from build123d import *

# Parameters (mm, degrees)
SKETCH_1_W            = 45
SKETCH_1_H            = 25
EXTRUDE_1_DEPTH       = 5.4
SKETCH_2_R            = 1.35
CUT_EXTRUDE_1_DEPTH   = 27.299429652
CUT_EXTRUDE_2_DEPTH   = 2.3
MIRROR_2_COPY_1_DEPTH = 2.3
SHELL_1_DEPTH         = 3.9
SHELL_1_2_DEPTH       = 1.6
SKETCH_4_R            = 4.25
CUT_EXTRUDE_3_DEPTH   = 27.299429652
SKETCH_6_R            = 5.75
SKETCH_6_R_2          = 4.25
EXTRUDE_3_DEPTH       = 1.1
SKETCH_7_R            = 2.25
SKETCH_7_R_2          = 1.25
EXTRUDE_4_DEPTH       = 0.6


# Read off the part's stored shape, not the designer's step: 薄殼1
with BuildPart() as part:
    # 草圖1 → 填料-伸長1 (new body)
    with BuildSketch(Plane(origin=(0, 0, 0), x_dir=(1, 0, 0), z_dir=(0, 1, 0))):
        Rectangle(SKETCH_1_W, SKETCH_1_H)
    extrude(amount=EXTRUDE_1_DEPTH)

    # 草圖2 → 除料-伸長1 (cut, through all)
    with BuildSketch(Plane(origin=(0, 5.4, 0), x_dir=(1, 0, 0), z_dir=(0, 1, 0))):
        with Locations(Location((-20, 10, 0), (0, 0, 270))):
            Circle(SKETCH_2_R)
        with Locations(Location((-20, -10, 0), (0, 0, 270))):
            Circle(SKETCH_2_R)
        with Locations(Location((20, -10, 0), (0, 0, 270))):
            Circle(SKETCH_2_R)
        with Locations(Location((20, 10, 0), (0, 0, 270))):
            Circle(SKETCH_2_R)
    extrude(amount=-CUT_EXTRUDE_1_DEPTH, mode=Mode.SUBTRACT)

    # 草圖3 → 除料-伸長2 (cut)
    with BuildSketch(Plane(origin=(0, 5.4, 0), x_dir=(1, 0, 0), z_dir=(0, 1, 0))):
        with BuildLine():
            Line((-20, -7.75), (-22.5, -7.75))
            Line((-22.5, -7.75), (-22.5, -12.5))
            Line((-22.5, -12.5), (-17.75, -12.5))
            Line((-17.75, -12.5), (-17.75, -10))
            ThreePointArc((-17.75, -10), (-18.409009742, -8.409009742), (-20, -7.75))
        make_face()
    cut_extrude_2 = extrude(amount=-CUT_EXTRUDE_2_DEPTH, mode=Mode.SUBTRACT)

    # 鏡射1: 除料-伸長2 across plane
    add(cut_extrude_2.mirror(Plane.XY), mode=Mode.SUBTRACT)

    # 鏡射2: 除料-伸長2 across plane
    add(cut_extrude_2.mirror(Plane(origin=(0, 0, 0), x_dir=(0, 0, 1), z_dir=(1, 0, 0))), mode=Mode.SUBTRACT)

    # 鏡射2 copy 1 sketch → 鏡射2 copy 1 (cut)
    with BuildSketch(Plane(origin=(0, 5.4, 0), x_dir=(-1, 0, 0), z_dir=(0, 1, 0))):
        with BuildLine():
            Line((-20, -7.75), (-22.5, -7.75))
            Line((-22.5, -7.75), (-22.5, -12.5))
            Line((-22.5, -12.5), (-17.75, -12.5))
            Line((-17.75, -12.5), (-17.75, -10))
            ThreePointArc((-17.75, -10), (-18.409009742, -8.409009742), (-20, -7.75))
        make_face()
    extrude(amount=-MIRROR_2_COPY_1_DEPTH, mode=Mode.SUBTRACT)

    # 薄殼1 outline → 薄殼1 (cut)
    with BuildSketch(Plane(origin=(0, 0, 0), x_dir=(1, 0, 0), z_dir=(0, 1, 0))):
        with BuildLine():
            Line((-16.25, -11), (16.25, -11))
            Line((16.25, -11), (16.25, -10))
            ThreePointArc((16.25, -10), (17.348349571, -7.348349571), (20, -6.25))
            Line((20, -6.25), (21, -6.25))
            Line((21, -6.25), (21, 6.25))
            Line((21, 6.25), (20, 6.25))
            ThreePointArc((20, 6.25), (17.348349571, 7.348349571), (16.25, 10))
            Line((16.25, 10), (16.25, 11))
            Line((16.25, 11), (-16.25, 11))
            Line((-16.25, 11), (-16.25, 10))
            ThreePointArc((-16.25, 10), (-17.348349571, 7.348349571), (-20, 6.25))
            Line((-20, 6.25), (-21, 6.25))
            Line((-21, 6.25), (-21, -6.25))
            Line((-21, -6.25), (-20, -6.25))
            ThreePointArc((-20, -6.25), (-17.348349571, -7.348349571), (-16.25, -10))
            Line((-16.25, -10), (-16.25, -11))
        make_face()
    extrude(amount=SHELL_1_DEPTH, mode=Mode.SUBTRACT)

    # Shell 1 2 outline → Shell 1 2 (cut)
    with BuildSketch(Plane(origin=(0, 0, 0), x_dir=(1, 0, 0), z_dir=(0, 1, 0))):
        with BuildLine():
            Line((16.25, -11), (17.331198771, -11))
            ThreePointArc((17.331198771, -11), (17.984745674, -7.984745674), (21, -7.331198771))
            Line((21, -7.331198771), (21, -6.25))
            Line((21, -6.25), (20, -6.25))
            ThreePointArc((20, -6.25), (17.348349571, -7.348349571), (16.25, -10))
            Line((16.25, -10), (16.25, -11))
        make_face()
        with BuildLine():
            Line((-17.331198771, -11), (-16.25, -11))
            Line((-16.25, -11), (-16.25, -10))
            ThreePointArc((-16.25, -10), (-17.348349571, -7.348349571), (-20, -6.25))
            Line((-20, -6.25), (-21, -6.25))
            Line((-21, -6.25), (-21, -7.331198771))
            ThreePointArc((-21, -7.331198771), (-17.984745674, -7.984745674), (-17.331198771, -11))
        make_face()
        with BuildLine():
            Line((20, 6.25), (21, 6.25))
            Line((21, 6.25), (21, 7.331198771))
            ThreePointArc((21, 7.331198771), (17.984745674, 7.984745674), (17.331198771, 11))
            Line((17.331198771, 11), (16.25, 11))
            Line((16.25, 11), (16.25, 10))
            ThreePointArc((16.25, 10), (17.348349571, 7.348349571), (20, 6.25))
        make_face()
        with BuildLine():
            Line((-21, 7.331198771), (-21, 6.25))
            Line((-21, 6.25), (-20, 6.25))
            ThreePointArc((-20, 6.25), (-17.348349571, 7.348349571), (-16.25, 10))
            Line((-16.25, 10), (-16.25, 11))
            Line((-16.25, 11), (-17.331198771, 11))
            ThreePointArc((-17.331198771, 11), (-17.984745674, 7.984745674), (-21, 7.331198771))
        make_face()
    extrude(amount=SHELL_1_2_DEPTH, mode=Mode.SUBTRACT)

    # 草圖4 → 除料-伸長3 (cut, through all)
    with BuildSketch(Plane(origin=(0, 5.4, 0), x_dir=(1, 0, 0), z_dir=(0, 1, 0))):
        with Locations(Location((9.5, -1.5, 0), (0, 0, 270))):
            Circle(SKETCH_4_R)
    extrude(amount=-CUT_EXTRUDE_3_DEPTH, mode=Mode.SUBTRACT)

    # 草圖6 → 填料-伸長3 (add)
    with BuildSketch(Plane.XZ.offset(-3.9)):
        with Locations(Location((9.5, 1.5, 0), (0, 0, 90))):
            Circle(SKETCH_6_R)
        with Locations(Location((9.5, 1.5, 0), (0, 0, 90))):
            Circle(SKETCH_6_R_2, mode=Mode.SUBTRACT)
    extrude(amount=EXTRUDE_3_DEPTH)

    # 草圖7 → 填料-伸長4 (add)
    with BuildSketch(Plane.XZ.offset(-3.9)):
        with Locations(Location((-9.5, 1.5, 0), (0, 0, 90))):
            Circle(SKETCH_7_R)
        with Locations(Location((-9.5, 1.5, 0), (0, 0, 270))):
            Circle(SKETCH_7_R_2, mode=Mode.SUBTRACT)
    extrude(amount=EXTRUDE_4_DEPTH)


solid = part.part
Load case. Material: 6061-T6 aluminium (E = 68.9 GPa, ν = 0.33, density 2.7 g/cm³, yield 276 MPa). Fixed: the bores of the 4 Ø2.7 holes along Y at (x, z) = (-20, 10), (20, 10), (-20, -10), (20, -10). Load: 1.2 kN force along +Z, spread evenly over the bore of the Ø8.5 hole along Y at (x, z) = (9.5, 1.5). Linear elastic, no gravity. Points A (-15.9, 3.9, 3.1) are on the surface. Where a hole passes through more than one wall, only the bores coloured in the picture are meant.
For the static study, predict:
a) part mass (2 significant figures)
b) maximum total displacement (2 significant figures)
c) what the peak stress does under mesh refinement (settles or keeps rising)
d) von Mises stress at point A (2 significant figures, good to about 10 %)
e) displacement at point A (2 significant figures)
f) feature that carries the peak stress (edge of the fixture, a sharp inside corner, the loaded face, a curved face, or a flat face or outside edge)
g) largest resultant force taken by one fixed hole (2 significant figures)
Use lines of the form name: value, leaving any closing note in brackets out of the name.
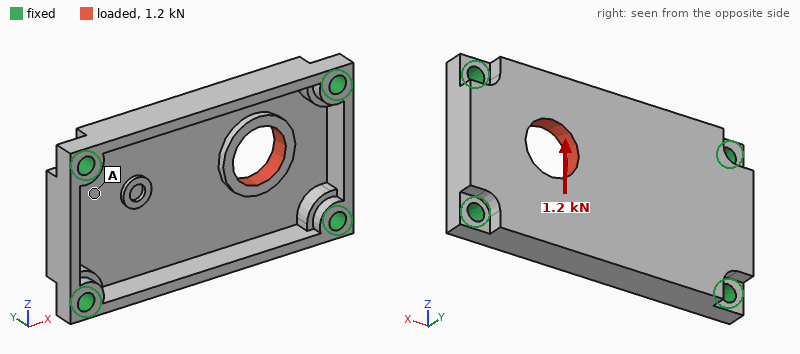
part mass: 6.6 g
maximum total displacement: 24 µm
what the peak stress does under mesh refinement: keeps rising
von Mises stress at point A: 23 MPa
displacement at point A: 5.0 µm
feature that carries the peak stress: edge of the fixture
largest resultant force taken by one fixed hole: 430 N
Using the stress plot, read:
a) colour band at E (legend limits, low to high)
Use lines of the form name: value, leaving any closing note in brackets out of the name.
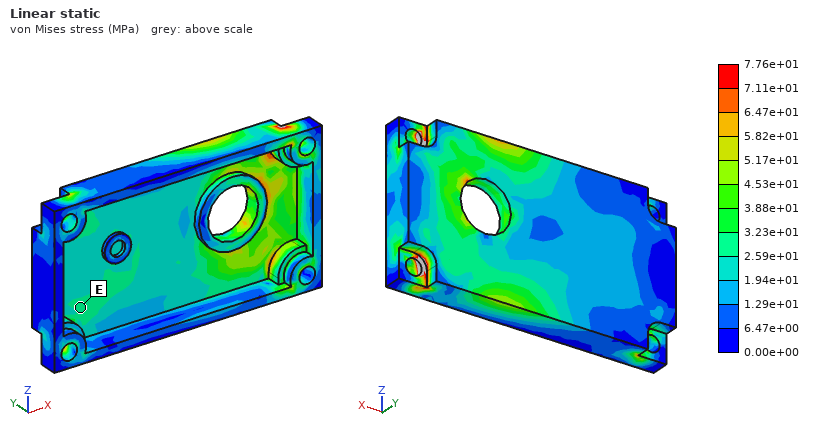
colour band at E: 2.59e+01 to 3.23e+01 MPa
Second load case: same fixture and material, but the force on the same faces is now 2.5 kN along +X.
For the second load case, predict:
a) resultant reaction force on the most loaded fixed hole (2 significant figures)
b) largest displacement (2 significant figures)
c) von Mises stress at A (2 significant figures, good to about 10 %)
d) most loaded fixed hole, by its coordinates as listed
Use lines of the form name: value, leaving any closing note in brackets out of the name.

resultant reaction force on the most loaded fixed hole: 850 N
largest displacement: 27 µm
von Mises stress at A: 17 MPa
most loaded fixed hole, by its coordinates as listed: (20, 10)
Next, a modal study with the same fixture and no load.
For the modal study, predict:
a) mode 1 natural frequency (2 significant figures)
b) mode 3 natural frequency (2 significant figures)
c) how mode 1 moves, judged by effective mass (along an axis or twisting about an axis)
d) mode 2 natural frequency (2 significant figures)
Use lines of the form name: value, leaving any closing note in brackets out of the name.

mode 1 natural frequency: 9200 Hz
mode 3 natural frequency: 18 kHz
how mode 1 moves, judged by effective mass: along Y
mode 2 natural frequency: 13 kHz
